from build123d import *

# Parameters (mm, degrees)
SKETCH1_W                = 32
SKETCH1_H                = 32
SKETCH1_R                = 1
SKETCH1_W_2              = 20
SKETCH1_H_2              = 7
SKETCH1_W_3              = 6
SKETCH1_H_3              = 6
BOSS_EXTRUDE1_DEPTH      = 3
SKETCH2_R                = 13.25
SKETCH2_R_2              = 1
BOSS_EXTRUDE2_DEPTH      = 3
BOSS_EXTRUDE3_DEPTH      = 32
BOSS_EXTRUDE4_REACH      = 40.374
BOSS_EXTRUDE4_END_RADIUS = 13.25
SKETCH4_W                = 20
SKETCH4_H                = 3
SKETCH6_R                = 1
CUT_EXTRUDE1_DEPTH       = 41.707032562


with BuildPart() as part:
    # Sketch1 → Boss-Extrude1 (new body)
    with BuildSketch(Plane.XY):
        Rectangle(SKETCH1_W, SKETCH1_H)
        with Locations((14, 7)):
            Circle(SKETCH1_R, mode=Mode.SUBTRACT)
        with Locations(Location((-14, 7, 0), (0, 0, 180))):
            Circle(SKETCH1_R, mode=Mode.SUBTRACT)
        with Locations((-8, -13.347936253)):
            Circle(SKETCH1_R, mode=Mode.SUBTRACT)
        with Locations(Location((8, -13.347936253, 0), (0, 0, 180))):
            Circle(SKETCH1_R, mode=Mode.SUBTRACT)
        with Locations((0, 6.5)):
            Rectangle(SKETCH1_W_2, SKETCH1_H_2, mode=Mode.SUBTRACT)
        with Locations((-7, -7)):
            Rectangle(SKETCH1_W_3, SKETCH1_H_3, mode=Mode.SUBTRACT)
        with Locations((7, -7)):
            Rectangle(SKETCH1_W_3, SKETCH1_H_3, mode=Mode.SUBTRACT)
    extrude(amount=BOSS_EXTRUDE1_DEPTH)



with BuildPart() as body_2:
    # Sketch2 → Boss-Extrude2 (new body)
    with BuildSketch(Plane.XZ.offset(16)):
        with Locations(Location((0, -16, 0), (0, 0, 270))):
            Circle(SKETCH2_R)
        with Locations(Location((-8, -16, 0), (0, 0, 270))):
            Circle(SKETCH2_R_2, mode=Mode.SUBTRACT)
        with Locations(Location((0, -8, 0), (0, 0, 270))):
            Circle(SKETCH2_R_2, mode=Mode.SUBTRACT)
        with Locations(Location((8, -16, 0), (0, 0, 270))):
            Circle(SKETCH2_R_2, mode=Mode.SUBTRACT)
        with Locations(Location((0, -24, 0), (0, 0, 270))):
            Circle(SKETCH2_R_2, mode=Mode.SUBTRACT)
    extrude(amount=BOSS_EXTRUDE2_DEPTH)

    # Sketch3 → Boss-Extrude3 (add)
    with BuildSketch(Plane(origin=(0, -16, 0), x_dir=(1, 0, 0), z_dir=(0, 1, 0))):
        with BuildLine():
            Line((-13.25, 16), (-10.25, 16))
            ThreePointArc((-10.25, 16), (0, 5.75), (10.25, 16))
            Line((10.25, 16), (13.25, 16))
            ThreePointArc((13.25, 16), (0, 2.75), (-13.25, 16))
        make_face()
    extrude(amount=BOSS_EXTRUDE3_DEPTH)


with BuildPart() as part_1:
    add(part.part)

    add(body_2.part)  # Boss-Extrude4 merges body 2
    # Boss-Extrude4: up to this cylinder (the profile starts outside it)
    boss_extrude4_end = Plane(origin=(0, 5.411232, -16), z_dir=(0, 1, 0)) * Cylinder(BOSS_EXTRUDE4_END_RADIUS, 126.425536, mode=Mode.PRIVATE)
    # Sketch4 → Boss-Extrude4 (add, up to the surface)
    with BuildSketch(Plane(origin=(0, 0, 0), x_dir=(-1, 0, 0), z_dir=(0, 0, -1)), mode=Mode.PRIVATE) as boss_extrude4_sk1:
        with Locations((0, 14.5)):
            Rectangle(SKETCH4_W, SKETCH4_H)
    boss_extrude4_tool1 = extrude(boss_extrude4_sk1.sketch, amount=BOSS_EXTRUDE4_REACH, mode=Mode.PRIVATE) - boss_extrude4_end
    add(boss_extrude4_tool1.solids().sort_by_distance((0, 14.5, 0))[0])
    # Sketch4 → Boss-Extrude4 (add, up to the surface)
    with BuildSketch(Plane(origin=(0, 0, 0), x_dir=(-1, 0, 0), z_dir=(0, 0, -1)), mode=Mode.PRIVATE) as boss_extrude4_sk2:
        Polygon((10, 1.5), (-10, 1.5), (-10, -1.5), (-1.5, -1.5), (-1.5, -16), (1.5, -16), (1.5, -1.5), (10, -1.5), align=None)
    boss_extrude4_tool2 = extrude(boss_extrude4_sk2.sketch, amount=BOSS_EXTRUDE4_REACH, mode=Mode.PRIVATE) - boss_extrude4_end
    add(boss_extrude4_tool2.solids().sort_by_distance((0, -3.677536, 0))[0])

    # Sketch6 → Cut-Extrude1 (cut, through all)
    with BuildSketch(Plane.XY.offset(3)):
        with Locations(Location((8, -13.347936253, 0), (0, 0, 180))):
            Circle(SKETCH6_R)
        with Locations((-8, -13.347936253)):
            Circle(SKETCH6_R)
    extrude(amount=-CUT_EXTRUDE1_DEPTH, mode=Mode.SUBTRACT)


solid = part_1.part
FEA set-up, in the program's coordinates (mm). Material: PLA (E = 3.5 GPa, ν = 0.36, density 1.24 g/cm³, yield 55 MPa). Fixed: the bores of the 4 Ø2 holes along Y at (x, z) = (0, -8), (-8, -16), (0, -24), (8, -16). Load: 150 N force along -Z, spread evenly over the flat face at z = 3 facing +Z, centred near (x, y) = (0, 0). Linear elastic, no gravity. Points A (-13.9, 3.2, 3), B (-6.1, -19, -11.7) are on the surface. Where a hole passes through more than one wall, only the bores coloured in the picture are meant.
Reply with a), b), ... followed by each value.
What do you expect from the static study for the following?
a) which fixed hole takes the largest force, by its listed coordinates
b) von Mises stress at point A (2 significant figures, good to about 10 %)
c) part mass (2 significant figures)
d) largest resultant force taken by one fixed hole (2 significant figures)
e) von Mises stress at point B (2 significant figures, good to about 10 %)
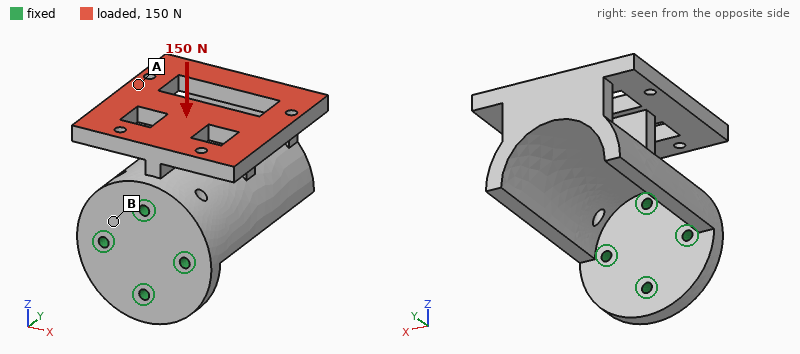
a) (0, -8)
b) 2.7 MPa
c) 10 g
d) 250 N
e) 6.3 MPa
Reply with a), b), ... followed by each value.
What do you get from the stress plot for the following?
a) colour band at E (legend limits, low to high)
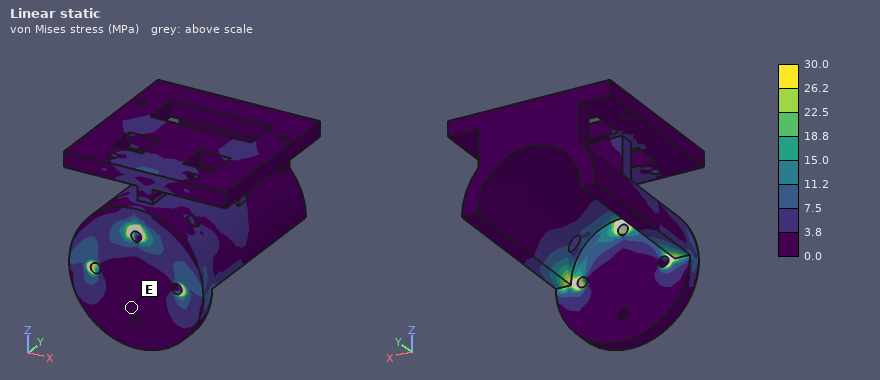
a) 0.0 to 3.8 MPa
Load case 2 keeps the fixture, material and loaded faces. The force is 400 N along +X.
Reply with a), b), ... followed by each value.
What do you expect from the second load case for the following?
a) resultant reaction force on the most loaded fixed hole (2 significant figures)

a) 400 N
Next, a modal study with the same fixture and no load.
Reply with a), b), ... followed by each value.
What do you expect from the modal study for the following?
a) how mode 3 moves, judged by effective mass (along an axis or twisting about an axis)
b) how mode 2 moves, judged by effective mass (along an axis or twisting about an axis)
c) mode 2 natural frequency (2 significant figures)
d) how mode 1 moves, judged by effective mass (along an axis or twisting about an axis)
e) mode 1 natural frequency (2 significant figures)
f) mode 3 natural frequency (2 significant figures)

a) along X
b) along X
c) 1200 Hz
d) along Z
e) 1100 Hz
f) 2100 Hz
